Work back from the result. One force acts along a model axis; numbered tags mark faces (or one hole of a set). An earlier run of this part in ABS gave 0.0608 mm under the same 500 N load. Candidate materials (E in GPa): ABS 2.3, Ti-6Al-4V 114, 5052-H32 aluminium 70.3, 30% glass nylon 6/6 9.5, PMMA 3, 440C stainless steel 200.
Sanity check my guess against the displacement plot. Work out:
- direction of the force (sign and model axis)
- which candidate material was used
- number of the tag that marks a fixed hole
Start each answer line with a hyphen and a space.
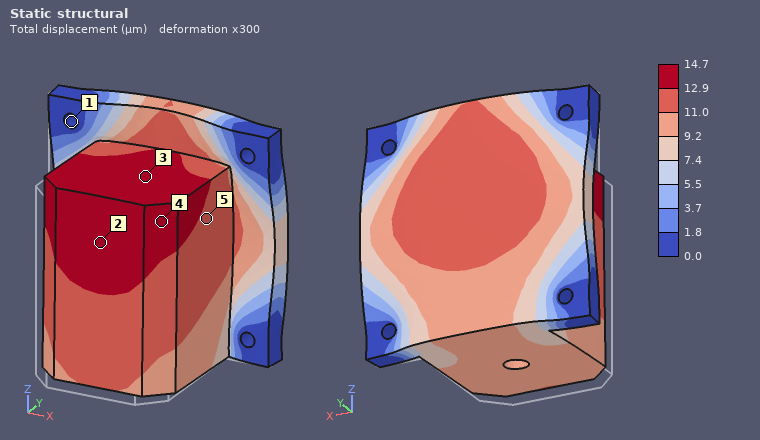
- +Y
- 30% glass nylon 6/6
- 1
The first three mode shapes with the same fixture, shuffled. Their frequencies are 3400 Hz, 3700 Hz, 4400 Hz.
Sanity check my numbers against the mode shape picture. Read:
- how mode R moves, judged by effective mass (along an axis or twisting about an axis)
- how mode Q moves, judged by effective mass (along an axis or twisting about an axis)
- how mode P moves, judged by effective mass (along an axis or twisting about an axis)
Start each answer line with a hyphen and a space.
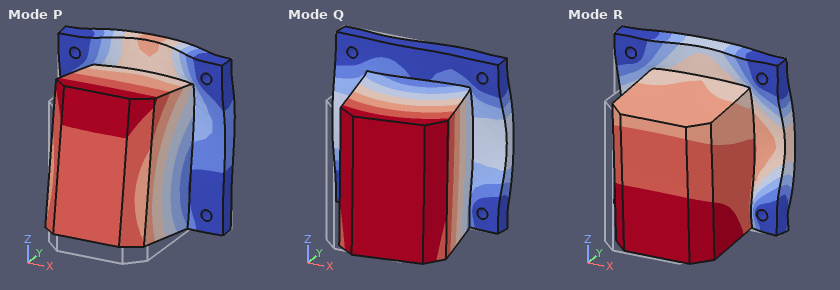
- along Y
- along X
- along Z
